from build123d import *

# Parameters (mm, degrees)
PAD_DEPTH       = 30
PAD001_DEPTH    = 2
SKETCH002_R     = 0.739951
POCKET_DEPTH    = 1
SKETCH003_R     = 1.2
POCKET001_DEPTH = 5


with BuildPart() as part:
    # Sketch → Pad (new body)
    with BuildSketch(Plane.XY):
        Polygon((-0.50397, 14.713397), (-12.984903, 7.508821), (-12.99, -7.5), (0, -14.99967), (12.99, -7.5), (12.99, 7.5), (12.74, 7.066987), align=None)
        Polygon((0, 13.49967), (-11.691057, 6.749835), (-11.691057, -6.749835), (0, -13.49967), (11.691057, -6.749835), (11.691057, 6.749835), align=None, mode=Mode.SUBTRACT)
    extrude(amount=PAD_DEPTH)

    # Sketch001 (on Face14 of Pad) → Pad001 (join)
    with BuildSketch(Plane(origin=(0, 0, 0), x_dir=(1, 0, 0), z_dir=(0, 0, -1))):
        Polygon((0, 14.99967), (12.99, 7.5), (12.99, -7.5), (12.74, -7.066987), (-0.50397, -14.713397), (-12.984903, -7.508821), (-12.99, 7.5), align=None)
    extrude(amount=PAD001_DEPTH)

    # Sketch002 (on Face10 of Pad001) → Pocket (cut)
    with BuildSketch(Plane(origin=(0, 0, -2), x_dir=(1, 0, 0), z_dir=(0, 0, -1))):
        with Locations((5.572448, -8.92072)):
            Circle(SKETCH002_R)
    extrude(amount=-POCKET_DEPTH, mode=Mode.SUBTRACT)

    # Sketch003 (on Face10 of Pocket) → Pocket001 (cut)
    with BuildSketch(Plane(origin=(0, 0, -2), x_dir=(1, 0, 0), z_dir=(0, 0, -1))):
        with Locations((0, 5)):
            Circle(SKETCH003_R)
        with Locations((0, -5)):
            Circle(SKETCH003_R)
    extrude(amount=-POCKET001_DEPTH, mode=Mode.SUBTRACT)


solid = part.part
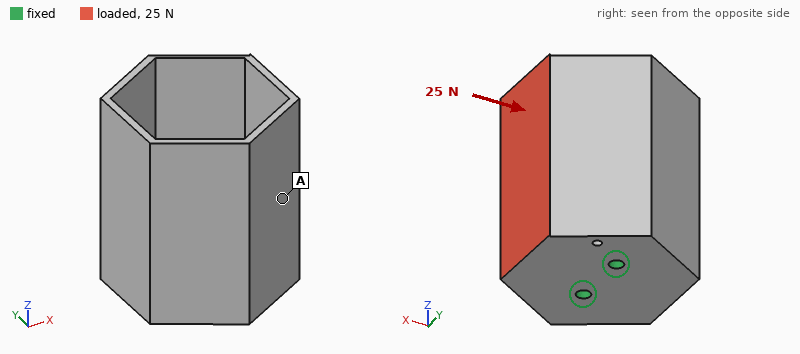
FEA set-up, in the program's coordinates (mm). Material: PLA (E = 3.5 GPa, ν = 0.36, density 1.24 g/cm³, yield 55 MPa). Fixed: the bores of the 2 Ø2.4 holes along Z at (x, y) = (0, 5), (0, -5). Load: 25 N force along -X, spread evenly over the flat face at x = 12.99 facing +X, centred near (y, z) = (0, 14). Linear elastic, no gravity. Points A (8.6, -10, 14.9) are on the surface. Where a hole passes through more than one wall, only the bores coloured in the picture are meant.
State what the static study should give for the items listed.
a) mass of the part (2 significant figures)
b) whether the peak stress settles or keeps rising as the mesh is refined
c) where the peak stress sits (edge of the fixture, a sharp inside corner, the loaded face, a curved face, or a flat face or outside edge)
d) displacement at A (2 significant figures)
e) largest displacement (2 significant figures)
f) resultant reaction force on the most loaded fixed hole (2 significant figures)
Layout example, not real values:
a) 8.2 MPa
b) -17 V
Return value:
a) 5.3 g
b) keeps rising
c) edge of the fixture
d) 0.23 mm
e) 0.51 mm
f) 13 N
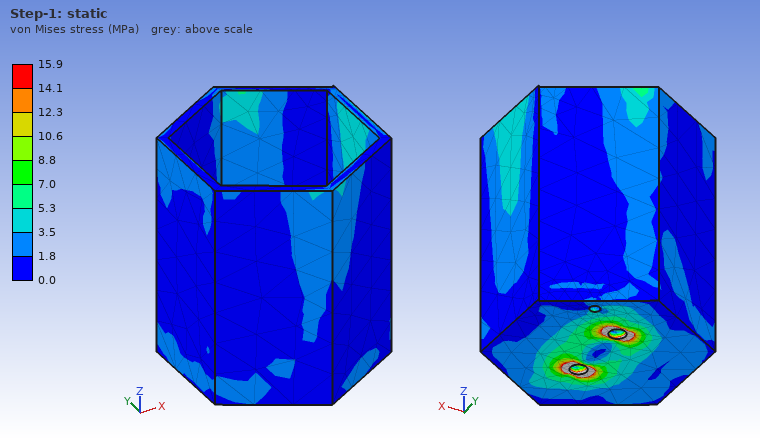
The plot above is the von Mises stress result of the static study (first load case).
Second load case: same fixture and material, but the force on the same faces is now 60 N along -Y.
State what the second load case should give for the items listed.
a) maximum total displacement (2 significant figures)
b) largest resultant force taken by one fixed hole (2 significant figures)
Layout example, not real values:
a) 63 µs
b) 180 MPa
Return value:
a) 0.52 mm
b) 94 N
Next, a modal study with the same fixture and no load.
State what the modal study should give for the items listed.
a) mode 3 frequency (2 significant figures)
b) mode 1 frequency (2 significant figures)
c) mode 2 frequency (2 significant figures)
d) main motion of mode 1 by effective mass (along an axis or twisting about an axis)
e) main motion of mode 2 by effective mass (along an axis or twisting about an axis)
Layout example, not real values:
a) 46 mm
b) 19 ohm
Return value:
a) 1600 Hz
b) 690 Hz
c) 1200 Hz
d) along X
e) along Y
